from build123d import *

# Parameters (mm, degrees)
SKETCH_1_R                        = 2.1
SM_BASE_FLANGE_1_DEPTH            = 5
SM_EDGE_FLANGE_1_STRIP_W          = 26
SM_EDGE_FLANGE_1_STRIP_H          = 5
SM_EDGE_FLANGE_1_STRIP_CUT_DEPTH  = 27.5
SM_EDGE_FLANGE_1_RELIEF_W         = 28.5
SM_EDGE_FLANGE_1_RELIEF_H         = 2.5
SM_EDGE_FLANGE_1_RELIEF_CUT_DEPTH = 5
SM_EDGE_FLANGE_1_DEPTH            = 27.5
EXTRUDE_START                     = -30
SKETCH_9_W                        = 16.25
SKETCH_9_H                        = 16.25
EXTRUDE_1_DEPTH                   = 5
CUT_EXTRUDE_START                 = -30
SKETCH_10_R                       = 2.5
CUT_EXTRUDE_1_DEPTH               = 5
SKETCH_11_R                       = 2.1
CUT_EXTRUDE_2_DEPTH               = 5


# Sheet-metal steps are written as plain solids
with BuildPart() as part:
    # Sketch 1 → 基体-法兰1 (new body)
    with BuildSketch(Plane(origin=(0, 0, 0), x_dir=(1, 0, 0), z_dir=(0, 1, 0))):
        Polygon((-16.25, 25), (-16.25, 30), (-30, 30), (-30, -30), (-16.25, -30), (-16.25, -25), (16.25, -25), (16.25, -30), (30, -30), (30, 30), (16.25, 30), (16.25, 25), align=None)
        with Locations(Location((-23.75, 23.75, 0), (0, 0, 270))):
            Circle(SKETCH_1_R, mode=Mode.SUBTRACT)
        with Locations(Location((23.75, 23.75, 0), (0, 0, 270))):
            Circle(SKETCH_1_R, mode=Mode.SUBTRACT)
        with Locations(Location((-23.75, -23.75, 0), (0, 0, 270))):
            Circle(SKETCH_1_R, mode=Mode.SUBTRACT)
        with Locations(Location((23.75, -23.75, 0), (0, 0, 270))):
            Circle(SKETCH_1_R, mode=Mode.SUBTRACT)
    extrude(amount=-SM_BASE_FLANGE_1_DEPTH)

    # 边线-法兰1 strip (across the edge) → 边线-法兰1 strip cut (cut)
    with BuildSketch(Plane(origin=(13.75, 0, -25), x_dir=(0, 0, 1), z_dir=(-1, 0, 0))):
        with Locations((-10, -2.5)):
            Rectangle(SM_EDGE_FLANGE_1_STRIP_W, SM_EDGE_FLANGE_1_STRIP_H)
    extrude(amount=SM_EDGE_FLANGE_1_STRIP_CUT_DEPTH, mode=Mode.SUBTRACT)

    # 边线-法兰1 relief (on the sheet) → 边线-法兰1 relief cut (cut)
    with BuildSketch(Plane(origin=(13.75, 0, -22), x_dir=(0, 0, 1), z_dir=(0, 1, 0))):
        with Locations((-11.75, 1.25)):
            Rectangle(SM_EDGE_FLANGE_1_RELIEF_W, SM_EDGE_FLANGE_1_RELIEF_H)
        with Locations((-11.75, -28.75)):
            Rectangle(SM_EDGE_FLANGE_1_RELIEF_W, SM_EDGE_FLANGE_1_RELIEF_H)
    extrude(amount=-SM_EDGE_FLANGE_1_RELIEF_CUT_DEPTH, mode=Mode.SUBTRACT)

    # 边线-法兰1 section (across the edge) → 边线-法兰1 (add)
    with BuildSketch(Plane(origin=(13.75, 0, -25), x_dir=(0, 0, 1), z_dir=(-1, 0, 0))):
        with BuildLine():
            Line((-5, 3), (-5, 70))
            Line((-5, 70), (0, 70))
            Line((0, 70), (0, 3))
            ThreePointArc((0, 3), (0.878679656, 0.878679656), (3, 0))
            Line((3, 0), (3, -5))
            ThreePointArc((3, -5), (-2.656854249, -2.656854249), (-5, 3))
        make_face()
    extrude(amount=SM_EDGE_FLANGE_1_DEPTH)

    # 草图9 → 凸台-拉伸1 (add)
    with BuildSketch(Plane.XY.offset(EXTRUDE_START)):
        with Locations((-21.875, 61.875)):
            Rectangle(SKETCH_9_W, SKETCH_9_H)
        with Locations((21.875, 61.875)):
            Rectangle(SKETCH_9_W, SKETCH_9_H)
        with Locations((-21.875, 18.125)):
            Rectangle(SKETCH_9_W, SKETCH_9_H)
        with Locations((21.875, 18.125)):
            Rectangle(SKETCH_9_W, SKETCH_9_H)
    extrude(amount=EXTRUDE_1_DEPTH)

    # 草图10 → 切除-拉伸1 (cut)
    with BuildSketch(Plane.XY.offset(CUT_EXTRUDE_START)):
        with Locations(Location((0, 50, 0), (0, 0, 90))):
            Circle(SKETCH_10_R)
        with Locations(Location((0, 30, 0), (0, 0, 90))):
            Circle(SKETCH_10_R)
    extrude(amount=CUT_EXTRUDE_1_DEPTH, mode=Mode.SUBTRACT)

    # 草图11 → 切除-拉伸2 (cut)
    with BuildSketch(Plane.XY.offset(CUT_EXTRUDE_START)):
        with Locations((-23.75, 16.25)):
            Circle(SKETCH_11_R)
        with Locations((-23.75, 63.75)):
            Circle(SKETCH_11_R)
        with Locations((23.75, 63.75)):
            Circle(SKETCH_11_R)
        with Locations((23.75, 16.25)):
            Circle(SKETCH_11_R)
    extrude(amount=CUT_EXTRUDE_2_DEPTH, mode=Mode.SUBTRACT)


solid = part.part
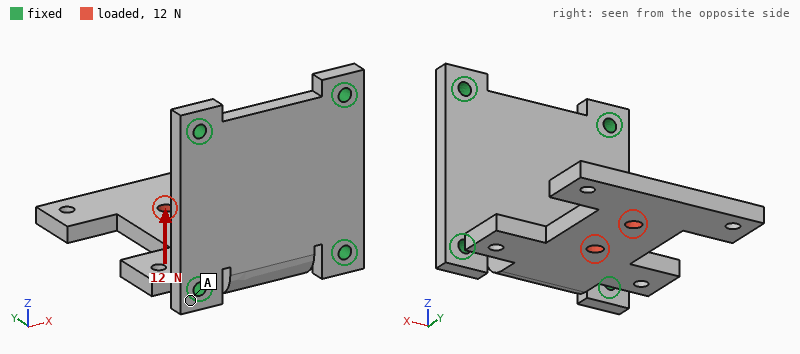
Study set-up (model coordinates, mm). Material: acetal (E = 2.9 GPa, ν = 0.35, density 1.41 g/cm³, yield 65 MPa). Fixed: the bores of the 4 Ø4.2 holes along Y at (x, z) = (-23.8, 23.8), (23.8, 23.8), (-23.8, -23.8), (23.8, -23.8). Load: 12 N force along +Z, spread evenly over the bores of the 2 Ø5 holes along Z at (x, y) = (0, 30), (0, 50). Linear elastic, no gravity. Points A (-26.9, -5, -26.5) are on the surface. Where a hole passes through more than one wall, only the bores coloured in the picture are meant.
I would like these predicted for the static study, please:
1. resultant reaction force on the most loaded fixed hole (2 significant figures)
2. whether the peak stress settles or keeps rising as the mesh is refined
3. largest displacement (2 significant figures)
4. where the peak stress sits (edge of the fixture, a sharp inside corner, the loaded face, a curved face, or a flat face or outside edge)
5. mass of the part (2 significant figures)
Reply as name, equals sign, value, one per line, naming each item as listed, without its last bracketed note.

resultant reaction force on the most loaded fixed hole = 7.1 N
whether the peak stress settles or keeps rising as the mesh is refined = keeps rising
largest displacement = 1.3 mm
where the peak stress sits = a sharp inside corner
mass of the part = 43 g
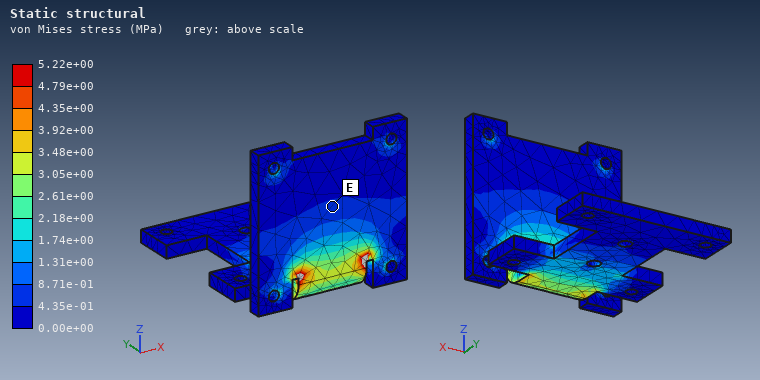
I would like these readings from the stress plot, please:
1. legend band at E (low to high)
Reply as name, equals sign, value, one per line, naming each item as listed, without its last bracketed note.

legend band at E = 4.35e-01 to 8.71e-01 MPa
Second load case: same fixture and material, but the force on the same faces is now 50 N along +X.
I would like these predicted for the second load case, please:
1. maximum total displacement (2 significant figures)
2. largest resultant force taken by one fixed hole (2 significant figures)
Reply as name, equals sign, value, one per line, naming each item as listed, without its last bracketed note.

maximum total displacement = 1.1 mm
largest resultant force taken by one fixed hole = 61 N
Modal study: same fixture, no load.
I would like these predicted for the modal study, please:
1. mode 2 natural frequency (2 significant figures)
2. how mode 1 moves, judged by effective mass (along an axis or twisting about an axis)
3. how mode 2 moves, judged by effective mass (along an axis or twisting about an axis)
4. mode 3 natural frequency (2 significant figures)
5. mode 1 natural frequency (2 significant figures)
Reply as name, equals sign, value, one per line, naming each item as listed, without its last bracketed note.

mode 2 natural frequency = 290 Hz
how mode 1 moves, judged by effective mass = along Z
how mode 2 moves, judged by effective mass = along X
mode 3 natural frequency = 470 Hz
mode 1 natural frequency = 130 Hz
